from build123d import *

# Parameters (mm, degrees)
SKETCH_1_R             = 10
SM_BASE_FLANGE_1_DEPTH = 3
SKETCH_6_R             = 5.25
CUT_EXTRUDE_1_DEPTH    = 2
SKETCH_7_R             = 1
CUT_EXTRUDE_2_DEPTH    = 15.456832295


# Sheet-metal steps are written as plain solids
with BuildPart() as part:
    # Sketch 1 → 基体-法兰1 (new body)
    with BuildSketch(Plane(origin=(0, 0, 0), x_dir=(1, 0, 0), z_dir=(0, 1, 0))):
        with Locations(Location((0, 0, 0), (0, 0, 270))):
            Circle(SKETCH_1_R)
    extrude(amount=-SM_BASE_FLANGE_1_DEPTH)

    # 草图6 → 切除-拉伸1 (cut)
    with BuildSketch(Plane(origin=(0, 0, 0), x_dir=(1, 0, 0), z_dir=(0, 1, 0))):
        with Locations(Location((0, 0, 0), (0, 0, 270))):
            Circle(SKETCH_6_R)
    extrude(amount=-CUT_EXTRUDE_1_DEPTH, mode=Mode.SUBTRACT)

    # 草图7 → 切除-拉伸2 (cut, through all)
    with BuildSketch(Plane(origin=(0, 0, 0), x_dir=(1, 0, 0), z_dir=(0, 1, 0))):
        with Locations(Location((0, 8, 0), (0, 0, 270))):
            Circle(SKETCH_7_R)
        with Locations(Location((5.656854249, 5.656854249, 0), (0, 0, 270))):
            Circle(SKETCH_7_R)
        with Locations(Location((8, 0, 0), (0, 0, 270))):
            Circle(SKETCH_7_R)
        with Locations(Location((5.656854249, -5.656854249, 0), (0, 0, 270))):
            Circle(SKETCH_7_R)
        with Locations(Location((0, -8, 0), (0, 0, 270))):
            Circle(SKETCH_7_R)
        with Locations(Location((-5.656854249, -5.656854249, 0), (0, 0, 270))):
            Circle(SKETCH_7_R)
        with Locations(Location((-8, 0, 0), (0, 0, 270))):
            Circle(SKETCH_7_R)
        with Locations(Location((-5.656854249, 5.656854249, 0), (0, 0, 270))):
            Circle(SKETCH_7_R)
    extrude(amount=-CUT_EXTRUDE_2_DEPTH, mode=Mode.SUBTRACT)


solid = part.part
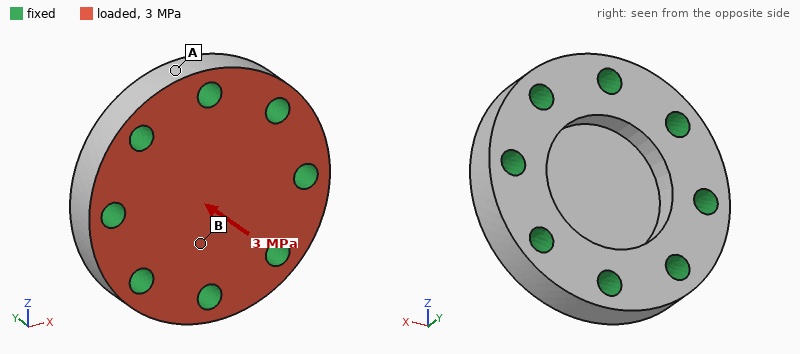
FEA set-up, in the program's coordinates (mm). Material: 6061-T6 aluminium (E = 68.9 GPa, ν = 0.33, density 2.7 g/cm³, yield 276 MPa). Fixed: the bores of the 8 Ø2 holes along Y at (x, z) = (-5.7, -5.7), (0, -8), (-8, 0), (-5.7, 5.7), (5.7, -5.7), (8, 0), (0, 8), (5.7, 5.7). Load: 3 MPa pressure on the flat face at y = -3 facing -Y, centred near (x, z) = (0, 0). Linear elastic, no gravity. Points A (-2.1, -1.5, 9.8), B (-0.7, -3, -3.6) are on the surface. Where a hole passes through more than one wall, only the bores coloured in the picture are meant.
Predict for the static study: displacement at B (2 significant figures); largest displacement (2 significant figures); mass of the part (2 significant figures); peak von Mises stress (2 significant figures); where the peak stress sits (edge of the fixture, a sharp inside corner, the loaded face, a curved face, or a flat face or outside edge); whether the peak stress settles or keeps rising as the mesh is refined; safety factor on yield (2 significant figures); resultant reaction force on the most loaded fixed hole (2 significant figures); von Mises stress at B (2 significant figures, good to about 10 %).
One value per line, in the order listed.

4.2 µm
9.7 µm
1.9 g
52 MPa
the loaded face
settles
5.3
110 N
21 MPa
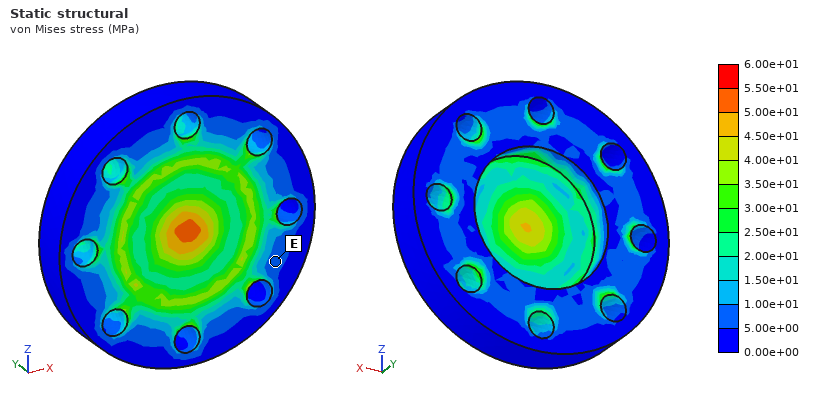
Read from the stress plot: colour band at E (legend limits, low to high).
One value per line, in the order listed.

5.00e+00 to 1.00e+01 MPa
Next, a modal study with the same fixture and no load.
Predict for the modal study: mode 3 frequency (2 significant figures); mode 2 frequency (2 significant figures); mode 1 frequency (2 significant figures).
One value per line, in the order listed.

130 kHz
130 kHz
68 kHz
